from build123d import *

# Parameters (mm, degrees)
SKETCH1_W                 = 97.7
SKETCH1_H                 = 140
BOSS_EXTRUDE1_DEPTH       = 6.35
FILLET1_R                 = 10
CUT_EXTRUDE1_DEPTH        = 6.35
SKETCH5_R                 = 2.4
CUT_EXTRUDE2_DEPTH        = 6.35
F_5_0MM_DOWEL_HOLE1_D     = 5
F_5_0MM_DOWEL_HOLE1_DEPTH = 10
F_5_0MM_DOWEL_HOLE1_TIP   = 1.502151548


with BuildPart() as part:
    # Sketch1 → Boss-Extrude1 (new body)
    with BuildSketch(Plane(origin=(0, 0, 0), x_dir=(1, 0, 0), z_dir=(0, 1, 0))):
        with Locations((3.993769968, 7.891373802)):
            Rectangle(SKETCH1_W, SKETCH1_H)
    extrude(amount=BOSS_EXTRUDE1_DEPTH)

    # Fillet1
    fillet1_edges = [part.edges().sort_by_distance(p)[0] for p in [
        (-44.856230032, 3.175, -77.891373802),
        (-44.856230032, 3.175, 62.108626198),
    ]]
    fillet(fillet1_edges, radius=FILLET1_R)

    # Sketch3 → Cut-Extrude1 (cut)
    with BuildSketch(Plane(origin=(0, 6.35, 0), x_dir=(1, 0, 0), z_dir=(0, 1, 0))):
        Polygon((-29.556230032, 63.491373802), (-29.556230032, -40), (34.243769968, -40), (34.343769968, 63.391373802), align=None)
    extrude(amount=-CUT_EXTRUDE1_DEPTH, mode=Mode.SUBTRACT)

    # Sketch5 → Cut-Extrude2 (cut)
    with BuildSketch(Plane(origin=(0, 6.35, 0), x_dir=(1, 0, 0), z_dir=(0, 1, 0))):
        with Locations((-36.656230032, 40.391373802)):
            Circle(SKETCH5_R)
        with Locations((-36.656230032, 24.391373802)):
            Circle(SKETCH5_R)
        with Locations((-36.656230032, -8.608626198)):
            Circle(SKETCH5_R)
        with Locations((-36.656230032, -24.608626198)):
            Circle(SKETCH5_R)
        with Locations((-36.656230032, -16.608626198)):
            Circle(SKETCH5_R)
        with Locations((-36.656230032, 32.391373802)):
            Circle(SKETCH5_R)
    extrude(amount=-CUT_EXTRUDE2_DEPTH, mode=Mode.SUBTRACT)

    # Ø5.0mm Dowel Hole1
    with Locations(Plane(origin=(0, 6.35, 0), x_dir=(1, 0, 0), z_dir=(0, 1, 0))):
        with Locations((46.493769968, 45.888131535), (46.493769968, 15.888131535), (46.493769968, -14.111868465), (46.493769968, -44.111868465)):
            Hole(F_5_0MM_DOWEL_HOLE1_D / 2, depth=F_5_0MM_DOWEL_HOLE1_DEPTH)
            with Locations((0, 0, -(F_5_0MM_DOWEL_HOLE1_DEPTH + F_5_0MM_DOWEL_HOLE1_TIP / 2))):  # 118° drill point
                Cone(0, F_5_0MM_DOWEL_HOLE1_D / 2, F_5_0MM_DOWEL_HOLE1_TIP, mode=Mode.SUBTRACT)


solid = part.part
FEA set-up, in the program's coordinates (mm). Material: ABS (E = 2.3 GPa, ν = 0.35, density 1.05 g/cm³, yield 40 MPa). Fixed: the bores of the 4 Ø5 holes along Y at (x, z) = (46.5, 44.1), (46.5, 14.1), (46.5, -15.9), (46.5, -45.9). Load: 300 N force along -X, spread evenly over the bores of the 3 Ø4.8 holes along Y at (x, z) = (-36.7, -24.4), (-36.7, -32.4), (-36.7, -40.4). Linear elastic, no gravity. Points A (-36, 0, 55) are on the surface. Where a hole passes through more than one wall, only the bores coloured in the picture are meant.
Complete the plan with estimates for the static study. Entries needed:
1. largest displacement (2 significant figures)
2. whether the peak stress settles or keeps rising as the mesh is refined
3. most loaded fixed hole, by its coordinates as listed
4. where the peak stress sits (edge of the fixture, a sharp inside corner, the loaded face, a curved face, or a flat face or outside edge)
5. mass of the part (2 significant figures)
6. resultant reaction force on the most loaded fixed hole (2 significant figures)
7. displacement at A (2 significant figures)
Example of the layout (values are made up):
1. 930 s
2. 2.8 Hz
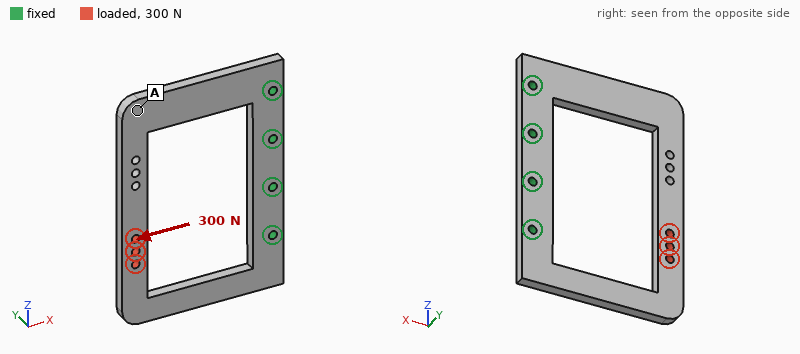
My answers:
1. 1.2 mm
2. keeps rising
3. (46.5, -45.9)
4. edge of the fixture
5. 46 g
6. 310 N
7. 0.21 mm
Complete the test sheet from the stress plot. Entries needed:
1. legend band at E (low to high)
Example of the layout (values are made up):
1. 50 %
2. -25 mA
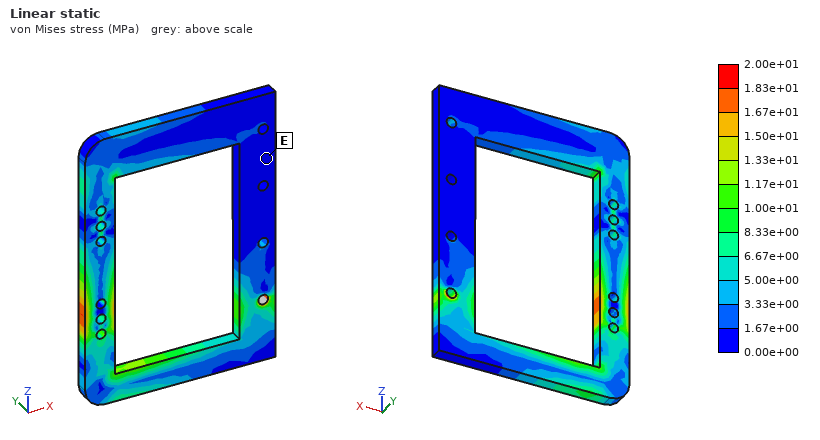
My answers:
1. 0.00e+00 to 1.67e+00 MPa
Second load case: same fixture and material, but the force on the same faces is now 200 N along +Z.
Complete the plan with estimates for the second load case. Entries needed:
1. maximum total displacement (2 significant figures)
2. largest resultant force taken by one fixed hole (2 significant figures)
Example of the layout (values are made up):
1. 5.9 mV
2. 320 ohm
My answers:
1. 1.8 mm
2. 270 N
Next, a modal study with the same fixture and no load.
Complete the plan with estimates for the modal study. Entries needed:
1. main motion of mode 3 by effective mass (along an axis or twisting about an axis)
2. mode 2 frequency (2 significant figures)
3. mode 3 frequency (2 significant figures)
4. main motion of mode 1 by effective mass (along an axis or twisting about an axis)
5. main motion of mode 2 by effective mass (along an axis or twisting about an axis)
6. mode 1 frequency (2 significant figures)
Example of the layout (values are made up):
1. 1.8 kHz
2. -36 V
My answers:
1. along Z
2. 210 Hz
3. 410 Hz
4. along Y
5. twisting about X
6. 110 Hz
